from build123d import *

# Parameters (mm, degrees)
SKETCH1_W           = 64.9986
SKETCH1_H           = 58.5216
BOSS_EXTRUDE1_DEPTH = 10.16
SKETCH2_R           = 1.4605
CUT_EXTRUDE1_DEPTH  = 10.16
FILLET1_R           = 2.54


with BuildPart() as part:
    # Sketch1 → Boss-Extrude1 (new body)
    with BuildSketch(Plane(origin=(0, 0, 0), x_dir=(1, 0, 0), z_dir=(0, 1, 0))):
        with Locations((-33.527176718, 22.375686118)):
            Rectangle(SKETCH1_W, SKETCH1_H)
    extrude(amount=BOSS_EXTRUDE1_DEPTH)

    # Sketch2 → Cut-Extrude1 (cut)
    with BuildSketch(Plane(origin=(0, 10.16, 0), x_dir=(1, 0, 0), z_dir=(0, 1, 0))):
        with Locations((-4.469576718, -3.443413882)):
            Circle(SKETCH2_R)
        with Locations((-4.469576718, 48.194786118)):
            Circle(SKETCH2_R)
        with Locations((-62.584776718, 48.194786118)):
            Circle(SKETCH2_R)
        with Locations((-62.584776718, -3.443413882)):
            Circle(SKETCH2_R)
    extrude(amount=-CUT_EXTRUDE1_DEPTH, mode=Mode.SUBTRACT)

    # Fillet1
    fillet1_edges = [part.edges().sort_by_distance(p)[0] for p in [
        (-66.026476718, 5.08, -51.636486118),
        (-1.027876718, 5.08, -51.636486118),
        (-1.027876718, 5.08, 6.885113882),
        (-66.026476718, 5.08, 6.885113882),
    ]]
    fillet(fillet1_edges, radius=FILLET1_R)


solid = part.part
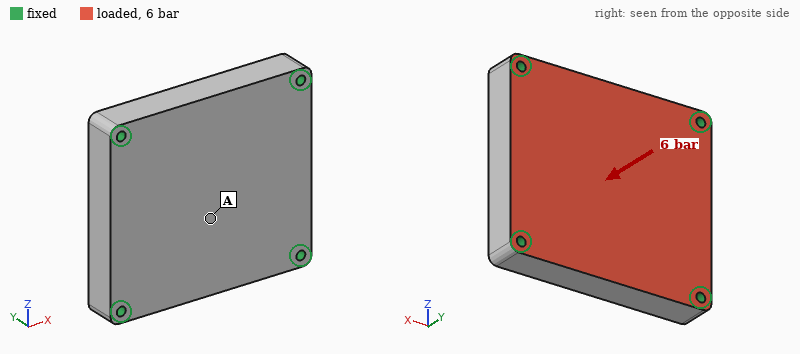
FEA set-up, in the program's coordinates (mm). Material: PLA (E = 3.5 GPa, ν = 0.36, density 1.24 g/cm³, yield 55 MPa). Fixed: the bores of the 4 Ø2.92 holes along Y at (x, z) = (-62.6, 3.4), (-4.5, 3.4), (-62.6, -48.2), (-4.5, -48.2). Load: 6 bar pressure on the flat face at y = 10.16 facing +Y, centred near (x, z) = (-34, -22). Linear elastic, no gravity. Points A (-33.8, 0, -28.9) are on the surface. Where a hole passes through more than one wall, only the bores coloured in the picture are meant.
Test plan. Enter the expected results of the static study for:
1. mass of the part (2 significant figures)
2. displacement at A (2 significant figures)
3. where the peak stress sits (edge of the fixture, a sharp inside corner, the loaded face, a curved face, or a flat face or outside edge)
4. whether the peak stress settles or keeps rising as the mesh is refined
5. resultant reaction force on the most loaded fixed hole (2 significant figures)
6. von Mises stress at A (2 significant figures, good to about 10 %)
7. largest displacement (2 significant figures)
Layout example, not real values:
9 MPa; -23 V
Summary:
48 g; 0.19 mm; edge of the fixture; keeps rising; 570 N; 6.8 MPa; 0.19 mm
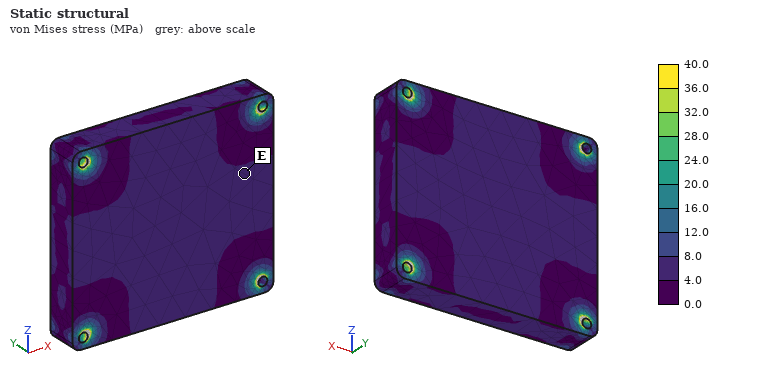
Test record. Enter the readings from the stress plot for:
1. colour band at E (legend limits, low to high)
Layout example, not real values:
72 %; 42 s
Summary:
4.0 to 8.0 MPa
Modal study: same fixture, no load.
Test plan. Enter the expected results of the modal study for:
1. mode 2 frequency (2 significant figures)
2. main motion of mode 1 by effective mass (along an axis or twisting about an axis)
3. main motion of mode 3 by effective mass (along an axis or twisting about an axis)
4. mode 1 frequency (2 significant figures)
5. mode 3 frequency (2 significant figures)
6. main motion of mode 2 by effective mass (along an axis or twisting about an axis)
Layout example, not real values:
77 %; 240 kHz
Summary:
4600 Hz; along Y; twisting about Z; 2900 Hz; 5100 Hz; twisting about X
